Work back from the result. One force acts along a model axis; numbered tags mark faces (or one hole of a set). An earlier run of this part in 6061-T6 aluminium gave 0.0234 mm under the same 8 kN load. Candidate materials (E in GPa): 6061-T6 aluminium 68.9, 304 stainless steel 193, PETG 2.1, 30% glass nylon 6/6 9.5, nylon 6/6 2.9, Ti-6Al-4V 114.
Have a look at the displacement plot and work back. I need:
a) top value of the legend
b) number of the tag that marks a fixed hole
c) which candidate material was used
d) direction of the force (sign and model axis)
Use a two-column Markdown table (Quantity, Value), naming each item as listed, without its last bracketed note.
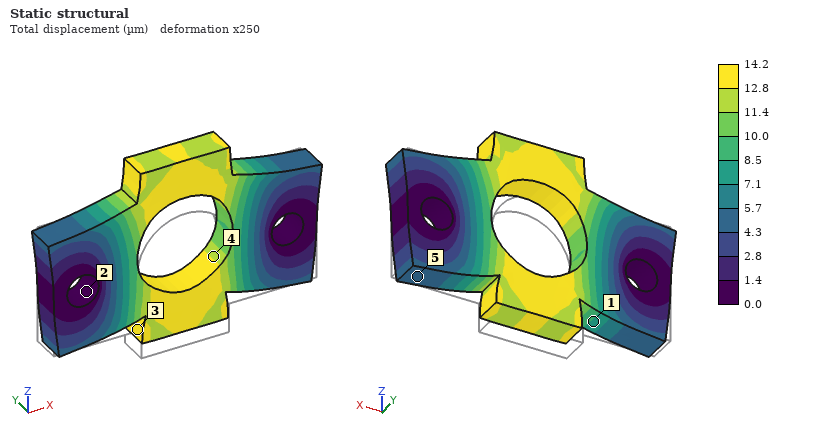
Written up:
| Quantity | Value |
|---|---|
| top value of the legend | 14.2 µm |
| number of the tag that marks a fixed hole | 2 |
| which candidate material was used | Ti-6Al-4V |
| direction of the force | +Z |
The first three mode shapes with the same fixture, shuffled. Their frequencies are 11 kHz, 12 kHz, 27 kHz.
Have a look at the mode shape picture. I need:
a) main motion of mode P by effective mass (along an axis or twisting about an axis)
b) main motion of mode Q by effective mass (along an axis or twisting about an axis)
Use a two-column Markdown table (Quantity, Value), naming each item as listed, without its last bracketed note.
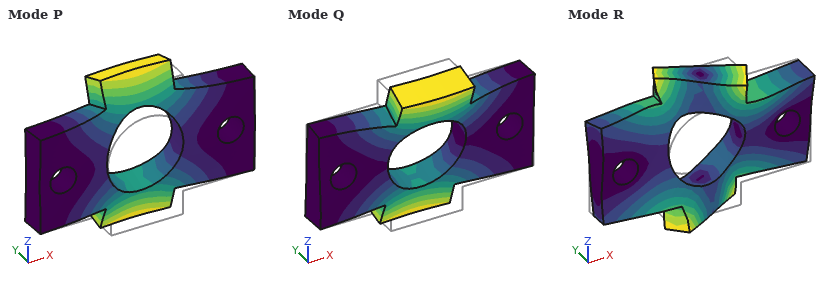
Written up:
| Quantity | Value |
|---|---|
| main motion of mode P by effective mass | along Y |
| main motion of mode Q by effective mass | twisting about X |
